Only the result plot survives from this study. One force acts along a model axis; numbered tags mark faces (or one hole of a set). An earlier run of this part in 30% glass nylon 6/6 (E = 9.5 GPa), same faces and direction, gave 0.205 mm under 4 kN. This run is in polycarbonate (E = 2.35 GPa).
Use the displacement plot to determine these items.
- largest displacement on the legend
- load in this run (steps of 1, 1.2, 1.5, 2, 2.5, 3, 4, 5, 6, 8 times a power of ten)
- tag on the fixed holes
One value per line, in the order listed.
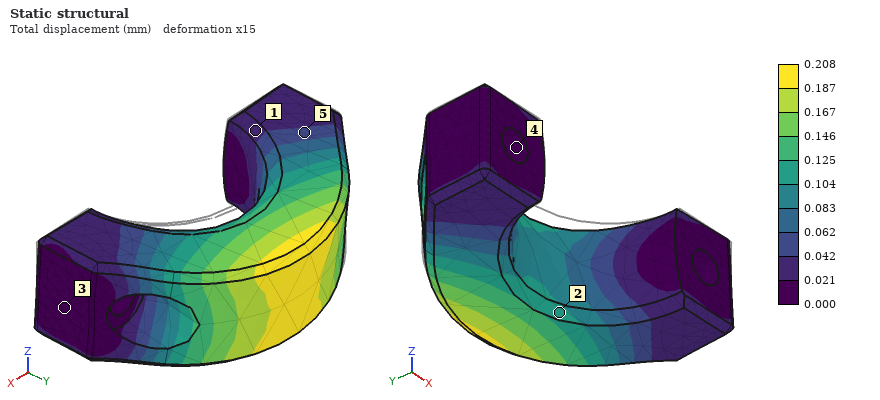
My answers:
0.208 mm
1 kN
4
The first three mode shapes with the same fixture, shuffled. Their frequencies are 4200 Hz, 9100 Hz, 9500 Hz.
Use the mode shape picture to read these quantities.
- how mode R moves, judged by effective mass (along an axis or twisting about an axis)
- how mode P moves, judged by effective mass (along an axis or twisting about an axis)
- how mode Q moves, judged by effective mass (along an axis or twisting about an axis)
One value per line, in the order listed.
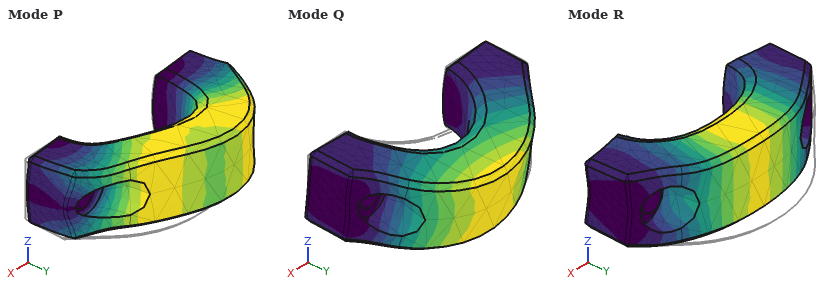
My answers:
along Y
along X
along Z
